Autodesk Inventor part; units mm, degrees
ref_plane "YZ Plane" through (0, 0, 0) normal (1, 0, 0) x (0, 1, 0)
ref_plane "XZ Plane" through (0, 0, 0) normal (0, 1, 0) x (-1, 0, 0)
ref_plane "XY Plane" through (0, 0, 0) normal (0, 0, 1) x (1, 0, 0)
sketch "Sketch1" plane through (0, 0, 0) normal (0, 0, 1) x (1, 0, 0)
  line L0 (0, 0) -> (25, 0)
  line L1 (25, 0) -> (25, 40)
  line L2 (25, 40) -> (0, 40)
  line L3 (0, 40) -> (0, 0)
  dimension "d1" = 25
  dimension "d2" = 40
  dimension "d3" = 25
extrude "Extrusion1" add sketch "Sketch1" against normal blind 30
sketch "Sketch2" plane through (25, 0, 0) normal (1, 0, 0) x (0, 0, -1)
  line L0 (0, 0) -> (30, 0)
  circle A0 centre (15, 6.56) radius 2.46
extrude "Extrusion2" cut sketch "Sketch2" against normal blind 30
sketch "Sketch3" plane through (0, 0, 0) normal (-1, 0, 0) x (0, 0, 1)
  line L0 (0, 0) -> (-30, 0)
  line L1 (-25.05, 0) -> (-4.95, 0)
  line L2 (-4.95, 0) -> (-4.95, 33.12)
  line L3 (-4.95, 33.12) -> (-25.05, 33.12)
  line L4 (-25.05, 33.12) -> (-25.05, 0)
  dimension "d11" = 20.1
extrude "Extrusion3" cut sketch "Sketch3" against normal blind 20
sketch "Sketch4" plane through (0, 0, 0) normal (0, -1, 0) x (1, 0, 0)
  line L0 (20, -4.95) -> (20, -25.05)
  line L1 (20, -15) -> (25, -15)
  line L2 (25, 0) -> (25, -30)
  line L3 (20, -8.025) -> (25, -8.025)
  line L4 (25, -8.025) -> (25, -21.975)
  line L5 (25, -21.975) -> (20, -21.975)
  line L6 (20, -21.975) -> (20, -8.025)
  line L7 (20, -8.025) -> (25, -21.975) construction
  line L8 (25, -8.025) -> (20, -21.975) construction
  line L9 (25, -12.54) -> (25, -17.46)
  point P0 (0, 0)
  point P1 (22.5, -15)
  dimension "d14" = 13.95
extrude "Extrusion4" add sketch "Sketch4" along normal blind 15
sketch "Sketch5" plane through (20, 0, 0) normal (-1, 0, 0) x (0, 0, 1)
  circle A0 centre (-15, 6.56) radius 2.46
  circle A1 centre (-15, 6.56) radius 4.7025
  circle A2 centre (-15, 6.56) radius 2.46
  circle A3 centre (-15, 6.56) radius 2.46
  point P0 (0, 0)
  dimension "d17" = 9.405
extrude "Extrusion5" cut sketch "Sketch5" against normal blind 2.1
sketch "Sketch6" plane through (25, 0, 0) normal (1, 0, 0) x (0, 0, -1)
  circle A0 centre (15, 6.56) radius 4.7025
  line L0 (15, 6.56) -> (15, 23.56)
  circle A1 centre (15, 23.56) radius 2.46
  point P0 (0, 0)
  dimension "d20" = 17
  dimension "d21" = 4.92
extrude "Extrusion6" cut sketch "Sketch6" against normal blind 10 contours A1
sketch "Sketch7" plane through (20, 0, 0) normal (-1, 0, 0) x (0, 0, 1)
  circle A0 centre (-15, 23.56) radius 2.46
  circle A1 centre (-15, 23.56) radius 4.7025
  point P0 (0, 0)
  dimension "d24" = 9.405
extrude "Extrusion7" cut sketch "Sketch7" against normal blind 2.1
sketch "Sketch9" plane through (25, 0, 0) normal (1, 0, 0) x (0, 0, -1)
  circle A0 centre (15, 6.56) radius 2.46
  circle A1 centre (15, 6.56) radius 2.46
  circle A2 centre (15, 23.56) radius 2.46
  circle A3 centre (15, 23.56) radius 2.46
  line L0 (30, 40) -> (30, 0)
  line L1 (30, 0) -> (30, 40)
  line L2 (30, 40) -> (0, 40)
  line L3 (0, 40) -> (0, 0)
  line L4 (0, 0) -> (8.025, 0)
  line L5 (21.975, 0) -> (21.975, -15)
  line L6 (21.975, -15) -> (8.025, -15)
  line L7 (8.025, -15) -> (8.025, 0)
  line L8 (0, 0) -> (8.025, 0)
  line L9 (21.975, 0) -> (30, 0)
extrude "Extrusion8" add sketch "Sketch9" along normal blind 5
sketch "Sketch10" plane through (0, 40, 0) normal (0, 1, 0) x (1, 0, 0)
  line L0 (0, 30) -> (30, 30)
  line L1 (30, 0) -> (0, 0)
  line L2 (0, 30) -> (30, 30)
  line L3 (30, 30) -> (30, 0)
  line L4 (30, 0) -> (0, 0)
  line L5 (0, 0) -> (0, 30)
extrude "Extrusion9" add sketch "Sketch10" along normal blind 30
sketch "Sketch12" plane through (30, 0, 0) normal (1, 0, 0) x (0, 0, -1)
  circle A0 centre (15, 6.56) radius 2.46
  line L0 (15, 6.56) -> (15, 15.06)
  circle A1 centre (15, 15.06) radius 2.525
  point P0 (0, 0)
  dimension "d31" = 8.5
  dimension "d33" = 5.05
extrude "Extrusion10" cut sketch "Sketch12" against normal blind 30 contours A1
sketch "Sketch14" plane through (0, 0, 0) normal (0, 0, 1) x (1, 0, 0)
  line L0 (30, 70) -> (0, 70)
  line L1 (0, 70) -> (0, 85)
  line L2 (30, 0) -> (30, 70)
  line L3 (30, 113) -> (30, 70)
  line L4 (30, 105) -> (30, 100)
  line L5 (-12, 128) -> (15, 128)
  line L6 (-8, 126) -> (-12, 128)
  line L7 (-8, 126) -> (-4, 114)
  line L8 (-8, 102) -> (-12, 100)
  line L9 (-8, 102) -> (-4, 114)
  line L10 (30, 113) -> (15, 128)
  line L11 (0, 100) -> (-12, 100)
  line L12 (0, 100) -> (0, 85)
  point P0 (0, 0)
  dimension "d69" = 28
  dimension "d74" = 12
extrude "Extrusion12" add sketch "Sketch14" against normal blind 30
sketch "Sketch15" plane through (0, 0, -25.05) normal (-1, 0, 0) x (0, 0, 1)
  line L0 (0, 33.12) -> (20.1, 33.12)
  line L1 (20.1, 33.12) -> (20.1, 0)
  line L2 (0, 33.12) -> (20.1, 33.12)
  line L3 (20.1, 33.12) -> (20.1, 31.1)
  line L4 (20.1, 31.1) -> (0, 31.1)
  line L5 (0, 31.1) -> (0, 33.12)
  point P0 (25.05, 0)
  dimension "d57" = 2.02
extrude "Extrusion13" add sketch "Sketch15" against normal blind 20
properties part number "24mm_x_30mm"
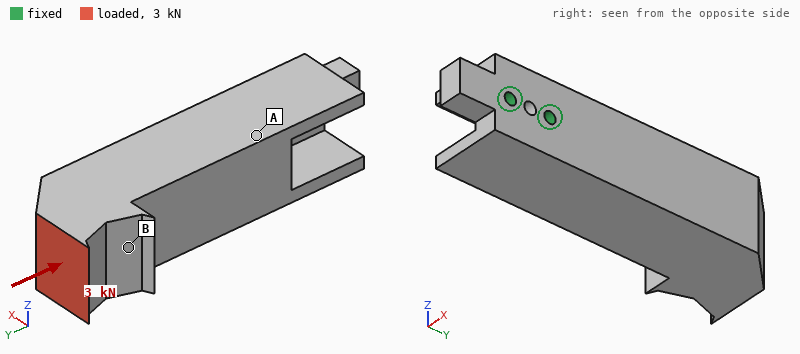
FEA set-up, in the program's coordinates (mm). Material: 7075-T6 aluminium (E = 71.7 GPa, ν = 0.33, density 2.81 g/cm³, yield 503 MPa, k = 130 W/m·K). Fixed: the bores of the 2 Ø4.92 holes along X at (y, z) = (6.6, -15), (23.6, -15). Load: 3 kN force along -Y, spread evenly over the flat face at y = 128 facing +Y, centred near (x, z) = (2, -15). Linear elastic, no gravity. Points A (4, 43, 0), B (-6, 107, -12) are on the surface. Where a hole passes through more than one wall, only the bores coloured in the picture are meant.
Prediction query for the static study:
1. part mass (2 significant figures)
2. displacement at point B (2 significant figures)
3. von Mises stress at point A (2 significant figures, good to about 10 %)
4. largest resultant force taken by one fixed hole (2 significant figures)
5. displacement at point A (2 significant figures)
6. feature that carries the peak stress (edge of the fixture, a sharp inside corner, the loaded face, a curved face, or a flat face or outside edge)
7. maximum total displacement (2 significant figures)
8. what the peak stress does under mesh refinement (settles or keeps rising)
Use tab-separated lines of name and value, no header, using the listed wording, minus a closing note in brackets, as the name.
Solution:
part mass	300 g
displacement at point B	0.17 mm
von Mises stress at point A	17 MPa
largest resultant force taken by one fixed hole	3.4 kN
displacement at point A	0.048 mm
feature that carries the peak stress	edge of the fixture
maximum total displacement	0.22 mm
what the peak stress does under mesh refinement	keeps rising
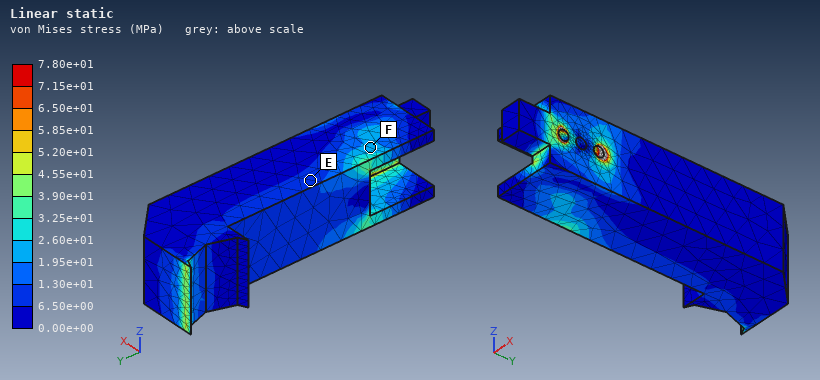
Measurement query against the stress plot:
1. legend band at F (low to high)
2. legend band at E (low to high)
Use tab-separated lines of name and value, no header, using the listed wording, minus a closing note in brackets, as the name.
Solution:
legend band at F	1.95e+01 to 2.60e+01 MPa
legend band at E	6.50e+00 to 1.30e+01 MPa
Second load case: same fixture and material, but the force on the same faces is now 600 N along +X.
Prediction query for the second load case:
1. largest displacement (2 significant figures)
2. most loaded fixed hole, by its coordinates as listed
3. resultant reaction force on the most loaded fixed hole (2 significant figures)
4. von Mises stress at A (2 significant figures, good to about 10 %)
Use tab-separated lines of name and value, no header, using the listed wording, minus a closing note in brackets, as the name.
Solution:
largest displacement	0.19 mm
most loaded fixed hole, by its coordinates as listed	(23.6, -15)
resultant reaction force on the most loaded fixed hole	3.1 kN
von Mises stress at A	14 MPa
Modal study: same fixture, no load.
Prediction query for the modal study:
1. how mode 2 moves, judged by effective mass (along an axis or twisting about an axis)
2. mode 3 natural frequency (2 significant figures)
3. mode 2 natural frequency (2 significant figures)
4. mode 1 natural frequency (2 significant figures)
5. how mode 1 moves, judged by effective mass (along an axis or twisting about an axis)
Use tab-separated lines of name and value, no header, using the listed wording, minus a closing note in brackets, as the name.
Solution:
how mode 2 moves, judged by effective mass	along Z
mode 3 natural frequency	3100 Hz
mode 2 natural frequency	1100 Hz
mode 1 natural frequency	960 Hz
how mode 1 moves, judged by effective mass	along X
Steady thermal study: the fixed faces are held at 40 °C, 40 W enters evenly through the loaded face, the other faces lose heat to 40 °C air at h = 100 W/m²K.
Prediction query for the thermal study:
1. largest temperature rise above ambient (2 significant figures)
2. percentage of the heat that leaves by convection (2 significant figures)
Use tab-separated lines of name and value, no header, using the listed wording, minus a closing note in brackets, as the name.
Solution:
largest temperature rise above ambient	36 K
percentage of the heat that leaves by convection	54 %
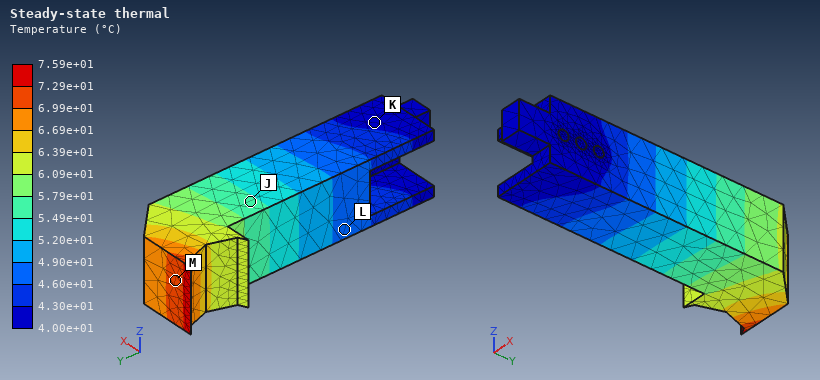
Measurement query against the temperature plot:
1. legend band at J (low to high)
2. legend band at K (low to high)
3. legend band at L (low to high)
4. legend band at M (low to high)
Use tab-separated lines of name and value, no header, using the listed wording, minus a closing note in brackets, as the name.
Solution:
legend band at J	5.49e+01 to 5.79e+01 °C
legend band at K	4.00e+01 to 4.30e+01 °C
legend band at L	4.60e+01 to 4.90e+01 °C
legend band at M	6.99e+01 to 7.29e+01 °C
